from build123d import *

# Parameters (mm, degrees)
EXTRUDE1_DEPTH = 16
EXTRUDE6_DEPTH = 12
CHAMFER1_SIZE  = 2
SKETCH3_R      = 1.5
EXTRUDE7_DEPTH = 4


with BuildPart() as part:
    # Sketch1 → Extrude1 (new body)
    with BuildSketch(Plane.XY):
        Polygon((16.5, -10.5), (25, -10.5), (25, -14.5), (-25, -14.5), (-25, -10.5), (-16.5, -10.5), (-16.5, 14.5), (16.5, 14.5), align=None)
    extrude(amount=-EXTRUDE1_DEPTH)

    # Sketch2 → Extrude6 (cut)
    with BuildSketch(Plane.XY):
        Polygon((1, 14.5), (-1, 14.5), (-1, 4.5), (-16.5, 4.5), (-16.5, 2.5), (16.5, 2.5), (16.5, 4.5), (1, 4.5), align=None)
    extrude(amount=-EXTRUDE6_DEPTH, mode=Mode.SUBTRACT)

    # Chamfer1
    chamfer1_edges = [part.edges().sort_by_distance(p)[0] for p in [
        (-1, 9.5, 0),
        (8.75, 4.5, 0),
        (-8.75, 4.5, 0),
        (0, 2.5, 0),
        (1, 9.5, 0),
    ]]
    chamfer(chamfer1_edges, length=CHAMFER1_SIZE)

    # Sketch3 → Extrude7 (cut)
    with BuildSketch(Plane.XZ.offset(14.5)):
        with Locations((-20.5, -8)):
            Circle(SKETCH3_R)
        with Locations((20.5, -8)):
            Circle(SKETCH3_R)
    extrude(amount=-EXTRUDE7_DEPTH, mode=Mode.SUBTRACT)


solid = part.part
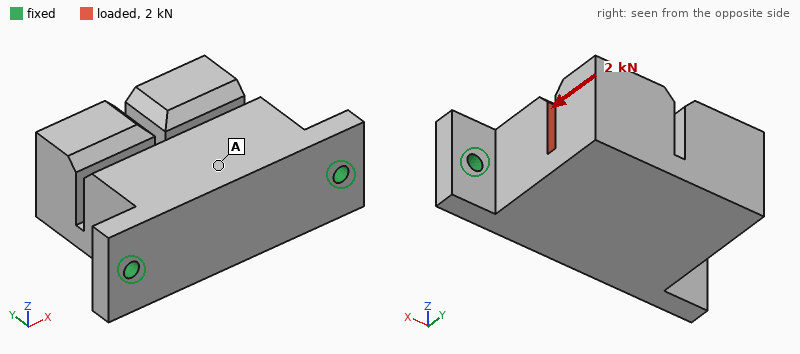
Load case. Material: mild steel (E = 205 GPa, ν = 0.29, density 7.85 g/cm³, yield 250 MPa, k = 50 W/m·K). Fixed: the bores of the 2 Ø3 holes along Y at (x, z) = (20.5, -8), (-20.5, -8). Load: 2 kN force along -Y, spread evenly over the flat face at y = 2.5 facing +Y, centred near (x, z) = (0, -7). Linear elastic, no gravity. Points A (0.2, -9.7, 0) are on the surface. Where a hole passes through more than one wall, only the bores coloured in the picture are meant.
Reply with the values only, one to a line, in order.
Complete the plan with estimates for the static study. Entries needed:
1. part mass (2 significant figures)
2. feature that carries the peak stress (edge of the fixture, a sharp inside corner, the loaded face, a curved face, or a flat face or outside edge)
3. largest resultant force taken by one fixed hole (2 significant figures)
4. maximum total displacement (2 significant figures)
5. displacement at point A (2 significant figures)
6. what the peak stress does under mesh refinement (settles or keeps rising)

120 g
edge of the fixture
1.1 kN
8.6 µm
5.7 µm
keeps rising
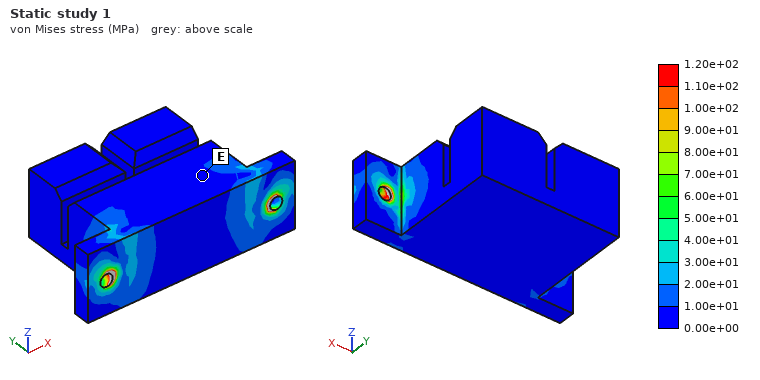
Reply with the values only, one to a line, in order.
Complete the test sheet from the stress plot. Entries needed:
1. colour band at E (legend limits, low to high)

0.00e+00 to 1.00e+01 MPa
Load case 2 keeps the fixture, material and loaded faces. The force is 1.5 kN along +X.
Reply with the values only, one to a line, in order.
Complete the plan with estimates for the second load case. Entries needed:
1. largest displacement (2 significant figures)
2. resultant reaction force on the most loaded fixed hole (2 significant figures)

4.1 µm
970 N
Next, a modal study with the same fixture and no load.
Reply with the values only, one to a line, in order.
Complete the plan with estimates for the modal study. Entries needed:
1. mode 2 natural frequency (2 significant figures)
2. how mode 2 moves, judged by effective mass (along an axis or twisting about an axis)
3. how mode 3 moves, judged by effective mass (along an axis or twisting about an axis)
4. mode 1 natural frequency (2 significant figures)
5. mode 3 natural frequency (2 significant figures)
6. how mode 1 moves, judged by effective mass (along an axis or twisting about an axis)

7800 Hz
along Y
along X
2700 Hz
9200 Hz
along Z
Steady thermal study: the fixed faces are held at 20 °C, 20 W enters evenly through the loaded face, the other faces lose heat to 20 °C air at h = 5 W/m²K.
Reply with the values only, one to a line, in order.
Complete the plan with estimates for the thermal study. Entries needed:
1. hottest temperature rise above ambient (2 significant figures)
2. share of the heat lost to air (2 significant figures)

38 K
3.4 %
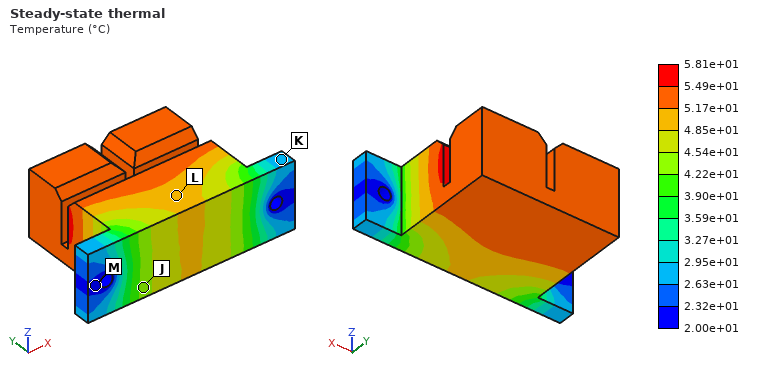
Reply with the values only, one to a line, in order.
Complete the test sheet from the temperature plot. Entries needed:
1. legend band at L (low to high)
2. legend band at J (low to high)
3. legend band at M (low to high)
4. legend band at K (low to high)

4.85e+01 to 5.17e+01 °C
4.22e+01 to 4.54e+01 °C
2.00e+01 to 2.32e+01 °C
2.63e+01 to 2.95e+01 °C
